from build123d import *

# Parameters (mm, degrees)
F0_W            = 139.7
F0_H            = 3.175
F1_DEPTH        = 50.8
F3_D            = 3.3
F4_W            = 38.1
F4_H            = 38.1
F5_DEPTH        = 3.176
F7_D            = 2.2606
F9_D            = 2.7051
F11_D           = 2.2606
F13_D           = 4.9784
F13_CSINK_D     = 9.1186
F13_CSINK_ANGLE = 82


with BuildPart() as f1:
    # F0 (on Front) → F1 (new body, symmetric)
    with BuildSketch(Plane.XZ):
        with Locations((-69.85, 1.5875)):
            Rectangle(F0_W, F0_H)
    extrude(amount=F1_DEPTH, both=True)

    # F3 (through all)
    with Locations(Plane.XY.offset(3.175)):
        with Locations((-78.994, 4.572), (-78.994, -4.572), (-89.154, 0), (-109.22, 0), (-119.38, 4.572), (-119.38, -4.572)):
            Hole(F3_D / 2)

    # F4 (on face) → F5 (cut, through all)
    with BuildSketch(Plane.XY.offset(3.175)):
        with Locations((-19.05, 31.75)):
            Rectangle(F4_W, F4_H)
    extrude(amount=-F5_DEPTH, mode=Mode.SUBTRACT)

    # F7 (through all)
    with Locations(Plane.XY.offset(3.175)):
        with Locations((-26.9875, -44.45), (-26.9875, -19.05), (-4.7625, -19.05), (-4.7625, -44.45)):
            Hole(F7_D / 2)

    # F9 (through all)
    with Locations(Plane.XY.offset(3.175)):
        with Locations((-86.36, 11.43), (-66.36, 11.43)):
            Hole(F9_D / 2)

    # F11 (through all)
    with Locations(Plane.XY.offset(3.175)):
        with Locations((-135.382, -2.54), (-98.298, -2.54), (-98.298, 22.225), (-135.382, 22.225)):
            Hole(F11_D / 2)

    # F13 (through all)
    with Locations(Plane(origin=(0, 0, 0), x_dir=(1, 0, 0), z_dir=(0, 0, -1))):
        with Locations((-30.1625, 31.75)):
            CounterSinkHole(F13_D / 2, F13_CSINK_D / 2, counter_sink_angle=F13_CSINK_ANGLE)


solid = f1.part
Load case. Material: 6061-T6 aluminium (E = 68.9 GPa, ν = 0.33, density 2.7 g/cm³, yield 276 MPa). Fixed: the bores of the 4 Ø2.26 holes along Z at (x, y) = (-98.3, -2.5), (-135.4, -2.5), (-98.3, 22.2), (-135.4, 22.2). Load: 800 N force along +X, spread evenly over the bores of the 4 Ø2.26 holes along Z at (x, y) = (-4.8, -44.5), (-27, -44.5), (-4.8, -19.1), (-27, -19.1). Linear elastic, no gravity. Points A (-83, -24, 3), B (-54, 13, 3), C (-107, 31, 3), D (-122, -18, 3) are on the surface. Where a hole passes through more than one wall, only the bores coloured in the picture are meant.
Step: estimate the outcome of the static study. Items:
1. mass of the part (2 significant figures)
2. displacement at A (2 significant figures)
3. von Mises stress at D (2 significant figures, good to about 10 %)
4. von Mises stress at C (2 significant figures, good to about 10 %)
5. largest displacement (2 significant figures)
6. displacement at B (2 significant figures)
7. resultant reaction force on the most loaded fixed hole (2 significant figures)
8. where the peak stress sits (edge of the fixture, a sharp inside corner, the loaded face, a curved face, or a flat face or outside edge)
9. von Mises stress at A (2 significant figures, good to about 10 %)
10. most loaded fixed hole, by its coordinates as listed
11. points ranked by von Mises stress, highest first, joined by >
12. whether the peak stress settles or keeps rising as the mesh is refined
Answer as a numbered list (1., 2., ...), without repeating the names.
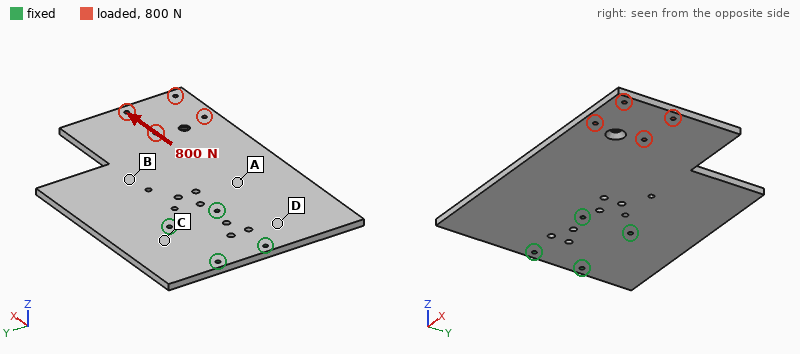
1. 110 g
2. 8.1 µm
3. 7.2 MPa
4. 2.7 MPa
5. 30 µm
6. 8.0 µm
7. 710 N
8. edge of the fixture
9. 5.1 MPa
10. (-98.3, -2.5)
11. D > A > C > B
12. keeps rising
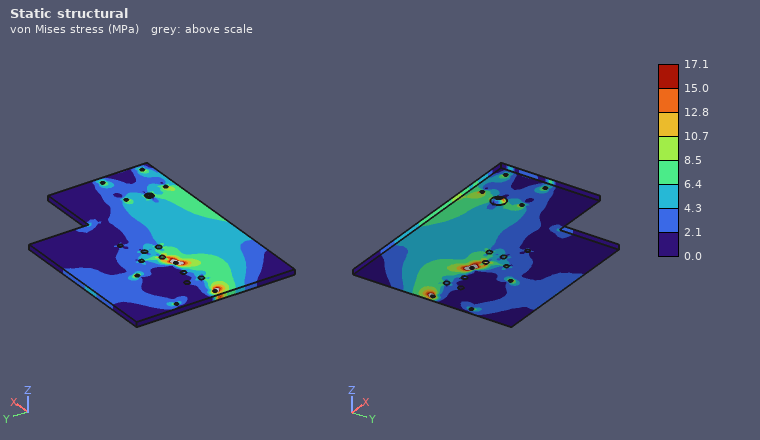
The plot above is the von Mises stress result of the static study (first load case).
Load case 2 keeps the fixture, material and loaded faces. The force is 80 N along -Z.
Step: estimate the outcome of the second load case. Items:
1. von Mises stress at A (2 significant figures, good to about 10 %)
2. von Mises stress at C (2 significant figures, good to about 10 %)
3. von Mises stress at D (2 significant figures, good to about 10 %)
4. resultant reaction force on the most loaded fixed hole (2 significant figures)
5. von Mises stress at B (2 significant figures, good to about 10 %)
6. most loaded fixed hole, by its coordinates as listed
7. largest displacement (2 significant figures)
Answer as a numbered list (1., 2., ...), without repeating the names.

1. 33 MPa
2. 9.2 MPa
3. 14 MPa
4. 210 N
5. 26 MPa
6. (-98.3, -2.5)
7. 1.8 mm
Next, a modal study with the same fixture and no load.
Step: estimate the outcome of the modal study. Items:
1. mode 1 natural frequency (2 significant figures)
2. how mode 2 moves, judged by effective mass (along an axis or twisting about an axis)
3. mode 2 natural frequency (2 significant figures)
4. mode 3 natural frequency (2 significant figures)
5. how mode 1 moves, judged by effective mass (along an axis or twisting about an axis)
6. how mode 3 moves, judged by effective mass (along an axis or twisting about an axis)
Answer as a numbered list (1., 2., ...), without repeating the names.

1. 280 Hz
2. twisting about X
3. 690 Hz
4. 1100 Hz
5. along Z
6. along Z
